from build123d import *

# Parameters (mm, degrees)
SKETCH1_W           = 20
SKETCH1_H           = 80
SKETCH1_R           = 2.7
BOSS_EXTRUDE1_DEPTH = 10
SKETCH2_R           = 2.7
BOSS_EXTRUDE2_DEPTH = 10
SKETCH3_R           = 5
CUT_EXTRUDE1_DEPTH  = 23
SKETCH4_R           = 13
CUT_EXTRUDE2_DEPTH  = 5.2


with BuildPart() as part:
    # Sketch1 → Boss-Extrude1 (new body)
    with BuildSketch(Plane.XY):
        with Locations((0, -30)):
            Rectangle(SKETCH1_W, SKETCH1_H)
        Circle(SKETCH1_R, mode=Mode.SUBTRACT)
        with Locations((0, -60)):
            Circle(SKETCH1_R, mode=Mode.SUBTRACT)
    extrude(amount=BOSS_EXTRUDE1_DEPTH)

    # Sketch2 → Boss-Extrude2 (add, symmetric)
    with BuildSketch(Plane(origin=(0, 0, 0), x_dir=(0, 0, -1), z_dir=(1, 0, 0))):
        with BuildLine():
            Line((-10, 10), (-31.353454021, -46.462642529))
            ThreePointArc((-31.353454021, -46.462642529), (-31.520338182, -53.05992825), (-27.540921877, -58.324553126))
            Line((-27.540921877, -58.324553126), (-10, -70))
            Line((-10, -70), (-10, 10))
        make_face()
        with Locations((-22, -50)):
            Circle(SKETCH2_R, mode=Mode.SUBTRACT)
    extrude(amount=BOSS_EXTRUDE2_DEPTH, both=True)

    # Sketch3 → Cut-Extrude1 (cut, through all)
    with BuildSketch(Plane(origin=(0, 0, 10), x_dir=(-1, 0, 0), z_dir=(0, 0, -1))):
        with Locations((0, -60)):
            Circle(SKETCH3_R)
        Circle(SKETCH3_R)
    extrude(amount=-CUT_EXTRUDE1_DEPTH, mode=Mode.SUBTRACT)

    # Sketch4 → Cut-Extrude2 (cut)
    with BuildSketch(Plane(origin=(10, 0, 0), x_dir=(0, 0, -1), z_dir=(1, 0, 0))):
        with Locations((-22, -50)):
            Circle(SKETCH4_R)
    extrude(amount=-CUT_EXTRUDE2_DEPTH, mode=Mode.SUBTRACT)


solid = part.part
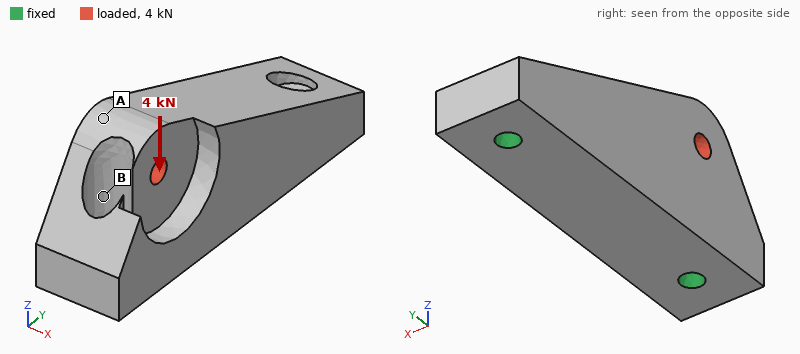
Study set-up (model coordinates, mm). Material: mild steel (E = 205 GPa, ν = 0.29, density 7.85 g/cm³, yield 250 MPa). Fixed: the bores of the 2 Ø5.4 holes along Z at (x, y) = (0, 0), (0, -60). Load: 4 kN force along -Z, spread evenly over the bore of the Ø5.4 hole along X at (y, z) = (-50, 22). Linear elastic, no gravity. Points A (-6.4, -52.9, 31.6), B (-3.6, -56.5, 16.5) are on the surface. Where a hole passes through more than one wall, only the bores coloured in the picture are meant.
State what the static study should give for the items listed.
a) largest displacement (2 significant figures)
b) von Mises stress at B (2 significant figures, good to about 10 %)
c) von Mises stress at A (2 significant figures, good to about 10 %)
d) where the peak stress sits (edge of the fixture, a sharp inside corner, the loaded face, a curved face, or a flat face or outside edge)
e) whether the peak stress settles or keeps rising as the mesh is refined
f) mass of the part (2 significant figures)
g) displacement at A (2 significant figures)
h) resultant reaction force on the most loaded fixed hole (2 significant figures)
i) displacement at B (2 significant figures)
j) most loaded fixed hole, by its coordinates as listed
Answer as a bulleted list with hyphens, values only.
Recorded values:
- 4.0 µm
- 29 MPa
- 10 MPa
- edge of the fixture
- keeps rising
- 240 g
- 3.6 µm
- 3.5 kN
- 2.6 µm
- (0, -60)
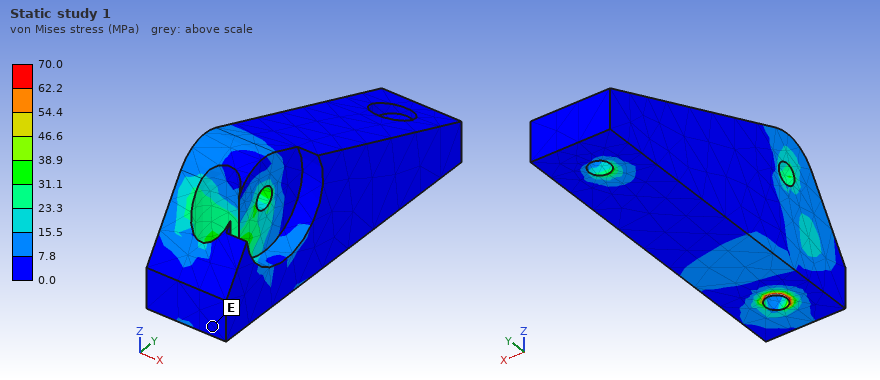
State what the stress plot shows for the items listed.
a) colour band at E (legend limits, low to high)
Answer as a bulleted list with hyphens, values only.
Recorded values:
- 0.0 to 7.8 MPa
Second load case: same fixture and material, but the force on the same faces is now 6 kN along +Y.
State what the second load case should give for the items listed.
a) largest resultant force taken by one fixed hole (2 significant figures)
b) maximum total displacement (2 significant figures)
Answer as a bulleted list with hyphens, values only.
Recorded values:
- 3.4 kN
- 5.7 µm
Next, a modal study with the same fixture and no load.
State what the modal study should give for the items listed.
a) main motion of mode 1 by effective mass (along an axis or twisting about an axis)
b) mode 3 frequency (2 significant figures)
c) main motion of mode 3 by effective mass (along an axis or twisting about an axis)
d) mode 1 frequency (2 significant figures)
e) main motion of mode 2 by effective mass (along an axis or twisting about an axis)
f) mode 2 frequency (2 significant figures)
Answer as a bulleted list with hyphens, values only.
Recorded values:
- along X
- 16 kHz
- along X
- 8500 Hz
- along Z
- 14 kHz
